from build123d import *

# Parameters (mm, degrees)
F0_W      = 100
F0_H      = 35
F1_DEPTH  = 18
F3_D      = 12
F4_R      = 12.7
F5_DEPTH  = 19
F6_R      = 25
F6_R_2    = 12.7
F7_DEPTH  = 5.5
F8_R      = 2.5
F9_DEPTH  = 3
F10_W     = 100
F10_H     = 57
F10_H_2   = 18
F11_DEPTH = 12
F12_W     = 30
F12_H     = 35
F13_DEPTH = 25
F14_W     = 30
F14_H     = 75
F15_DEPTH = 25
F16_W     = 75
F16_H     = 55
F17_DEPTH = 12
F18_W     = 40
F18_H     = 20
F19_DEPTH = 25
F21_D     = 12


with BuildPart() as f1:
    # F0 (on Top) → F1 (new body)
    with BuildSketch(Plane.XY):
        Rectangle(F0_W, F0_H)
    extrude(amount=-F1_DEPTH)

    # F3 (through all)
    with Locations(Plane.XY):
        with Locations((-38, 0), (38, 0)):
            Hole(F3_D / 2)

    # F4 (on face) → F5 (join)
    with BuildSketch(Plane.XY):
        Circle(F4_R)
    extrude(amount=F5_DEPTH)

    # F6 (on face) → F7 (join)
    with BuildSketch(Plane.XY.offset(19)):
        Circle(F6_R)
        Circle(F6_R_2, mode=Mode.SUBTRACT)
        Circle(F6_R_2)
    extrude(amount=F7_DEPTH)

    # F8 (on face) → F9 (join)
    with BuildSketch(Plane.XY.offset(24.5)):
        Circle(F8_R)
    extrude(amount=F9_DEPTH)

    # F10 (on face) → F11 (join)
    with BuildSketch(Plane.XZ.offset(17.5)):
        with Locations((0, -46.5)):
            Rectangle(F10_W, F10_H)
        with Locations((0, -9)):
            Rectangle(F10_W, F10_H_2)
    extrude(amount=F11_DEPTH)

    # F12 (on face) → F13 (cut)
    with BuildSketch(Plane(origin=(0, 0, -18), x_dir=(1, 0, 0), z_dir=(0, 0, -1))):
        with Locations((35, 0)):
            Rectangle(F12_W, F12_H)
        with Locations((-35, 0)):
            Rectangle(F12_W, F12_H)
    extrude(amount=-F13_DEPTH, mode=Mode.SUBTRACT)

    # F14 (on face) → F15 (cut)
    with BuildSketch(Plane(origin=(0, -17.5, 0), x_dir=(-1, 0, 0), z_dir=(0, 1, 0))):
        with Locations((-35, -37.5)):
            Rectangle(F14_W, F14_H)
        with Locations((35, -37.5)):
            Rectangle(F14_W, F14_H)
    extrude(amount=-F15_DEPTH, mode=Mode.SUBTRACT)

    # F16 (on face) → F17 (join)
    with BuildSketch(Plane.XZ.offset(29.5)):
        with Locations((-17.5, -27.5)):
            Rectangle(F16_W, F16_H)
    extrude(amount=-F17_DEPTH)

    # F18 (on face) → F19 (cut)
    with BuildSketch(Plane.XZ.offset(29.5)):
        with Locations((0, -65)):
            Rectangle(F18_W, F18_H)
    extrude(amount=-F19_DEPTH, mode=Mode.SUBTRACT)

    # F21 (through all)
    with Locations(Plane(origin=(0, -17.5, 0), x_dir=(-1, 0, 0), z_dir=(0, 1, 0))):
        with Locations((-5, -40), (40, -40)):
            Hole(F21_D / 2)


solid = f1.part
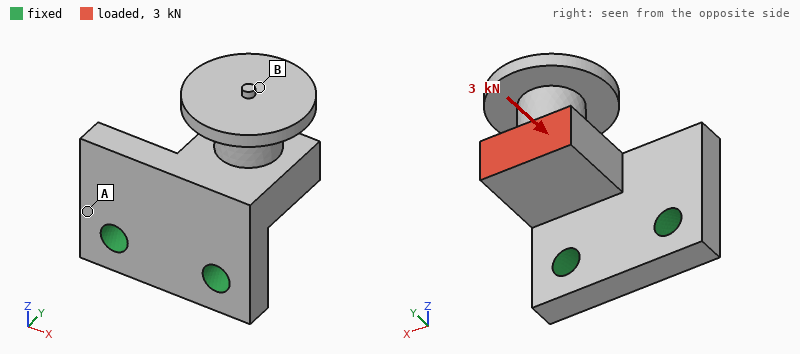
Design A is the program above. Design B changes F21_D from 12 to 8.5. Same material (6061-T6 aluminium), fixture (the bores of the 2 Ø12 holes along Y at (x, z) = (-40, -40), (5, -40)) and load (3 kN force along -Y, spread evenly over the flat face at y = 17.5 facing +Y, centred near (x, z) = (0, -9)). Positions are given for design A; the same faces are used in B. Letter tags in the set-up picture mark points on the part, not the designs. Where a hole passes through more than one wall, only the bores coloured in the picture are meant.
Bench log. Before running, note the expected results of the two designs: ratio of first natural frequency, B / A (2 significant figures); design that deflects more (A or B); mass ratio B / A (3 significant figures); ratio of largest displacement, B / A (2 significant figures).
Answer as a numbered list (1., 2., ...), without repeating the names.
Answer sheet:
1. 0.94
2. B
3. 1.01
4. 1.2
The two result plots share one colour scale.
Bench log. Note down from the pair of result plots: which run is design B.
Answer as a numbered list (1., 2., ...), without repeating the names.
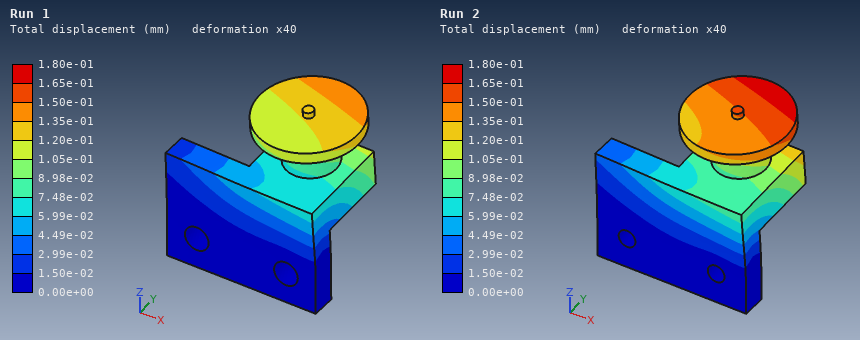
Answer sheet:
1. Run 2
